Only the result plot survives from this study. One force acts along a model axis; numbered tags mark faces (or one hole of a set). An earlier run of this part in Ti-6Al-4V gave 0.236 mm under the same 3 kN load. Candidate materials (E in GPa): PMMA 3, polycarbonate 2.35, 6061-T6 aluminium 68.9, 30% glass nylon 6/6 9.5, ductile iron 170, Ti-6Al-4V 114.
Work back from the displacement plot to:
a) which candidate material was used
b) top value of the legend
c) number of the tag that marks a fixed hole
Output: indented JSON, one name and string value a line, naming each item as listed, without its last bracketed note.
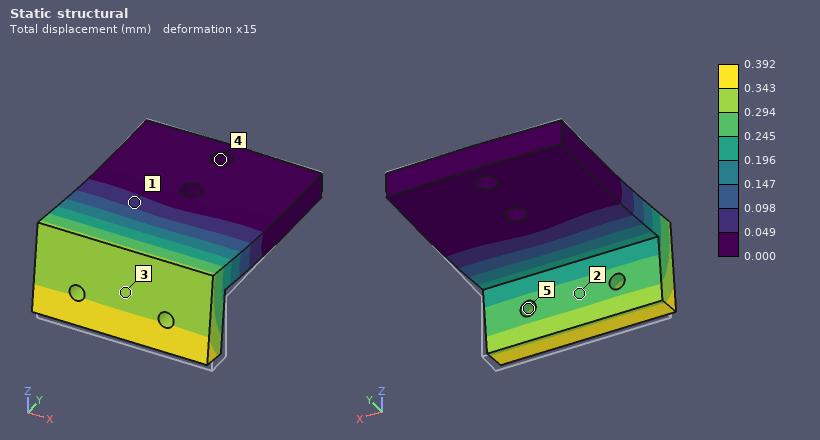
{
  "which candidate material was used": "6061-T6 aluminium",
  "top value of the legend": "0.392 mm",
  "number of the tag that marks a fixed hole": "4"
}
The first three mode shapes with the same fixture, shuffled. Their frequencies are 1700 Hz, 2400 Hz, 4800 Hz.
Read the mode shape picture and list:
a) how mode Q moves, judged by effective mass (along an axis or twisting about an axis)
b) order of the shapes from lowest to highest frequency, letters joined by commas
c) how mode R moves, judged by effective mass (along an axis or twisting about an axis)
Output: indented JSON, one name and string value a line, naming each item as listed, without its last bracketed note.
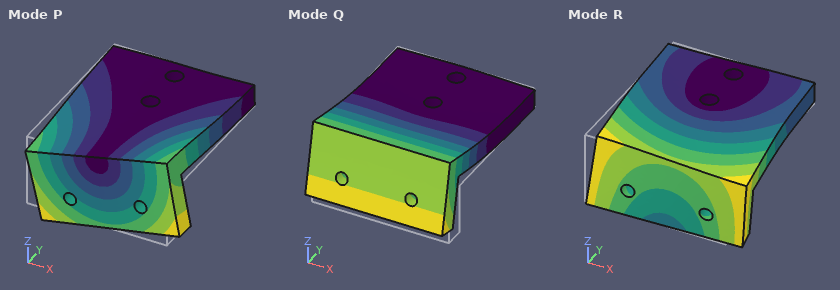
{
  "how mode Q moves, judged by effective mass": "along Z",
  "order of the shapes from lowest to highest frequency, letters joined by commas": "Q, P, R",
  "how mode R moves, judged by effective mass": "along X"
}
